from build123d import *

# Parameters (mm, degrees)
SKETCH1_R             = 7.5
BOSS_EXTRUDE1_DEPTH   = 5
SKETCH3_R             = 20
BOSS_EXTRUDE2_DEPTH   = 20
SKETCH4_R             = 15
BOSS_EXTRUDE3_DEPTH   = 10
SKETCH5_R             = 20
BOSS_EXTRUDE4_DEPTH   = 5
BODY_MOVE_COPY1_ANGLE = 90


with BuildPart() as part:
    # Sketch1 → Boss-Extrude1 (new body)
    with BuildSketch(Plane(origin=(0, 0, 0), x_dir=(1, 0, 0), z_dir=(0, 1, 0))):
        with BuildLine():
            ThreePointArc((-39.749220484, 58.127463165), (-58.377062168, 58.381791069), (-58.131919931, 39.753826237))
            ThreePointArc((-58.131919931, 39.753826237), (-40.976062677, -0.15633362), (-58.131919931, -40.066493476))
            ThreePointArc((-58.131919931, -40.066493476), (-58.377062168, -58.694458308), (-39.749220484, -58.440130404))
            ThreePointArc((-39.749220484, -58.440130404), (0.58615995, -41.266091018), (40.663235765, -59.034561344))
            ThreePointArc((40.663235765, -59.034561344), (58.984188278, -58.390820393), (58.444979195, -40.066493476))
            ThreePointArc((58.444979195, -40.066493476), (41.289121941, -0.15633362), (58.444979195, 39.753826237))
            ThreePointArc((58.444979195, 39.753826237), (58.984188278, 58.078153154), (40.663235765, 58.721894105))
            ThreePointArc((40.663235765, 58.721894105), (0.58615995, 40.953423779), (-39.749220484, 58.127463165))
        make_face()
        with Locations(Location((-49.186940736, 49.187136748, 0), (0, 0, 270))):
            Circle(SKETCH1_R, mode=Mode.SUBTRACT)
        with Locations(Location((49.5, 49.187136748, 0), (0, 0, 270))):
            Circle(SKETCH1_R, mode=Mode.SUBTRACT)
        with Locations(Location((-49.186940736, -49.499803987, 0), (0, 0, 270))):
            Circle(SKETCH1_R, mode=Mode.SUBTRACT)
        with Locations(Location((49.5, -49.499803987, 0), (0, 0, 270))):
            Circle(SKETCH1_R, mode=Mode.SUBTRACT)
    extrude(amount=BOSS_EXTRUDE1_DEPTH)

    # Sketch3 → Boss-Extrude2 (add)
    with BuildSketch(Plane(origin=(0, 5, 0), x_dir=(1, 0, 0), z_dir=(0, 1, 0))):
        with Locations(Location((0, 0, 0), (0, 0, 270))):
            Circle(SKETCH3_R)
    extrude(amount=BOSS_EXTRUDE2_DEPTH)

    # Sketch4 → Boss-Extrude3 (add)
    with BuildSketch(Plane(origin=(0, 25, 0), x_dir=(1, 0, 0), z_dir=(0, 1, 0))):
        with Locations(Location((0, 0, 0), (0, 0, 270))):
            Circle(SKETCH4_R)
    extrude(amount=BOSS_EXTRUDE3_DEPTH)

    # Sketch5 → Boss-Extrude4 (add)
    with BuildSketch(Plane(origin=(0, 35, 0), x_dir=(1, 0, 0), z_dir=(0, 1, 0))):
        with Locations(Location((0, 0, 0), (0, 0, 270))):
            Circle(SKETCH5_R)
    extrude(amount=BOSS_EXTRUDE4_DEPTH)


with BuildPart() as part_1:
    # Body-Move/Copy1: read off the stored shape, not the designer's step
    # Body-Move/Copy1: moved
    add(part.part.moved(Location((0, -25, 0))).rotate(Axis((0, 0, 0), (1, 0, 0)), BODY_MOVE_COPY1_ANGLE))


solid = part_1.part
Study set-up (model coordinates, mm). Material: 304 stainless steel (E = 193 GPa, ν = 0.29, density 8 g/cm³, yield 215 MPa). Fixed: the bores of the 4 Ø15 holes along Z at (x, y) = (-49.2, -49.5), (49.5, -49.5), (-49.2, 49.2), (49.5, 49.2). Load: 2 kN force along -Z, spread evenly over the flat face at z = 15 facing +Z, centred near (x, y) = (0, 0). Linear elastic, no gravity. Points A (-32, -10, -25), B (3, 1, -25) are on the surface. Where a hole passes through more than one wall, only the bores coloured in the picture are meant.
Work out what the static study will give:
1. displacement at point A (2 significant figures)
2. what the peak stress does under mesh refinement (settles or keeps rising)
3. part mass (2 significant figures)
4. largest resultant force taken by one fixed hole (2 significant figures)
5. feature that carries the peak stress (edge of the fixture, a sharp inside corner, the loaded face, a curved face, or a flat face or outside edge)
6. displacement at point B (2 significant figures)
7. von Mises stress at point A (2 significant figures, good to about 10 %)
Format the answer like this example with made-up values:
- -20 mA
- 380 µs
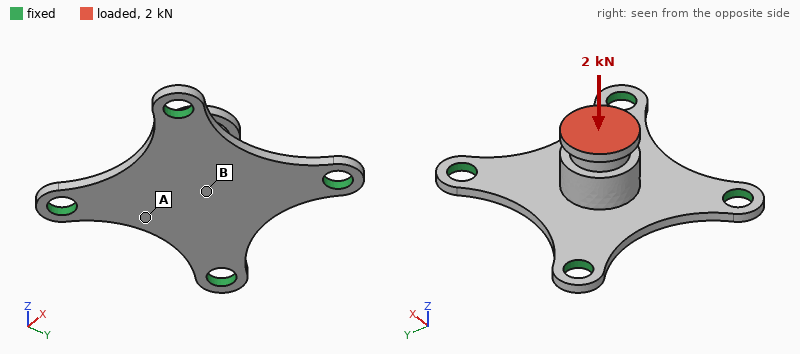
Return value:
- 46 µm
- keeps rising
- 690 g
- 530 N
- edge of the fixture
- 58 µm
- 30 MPa
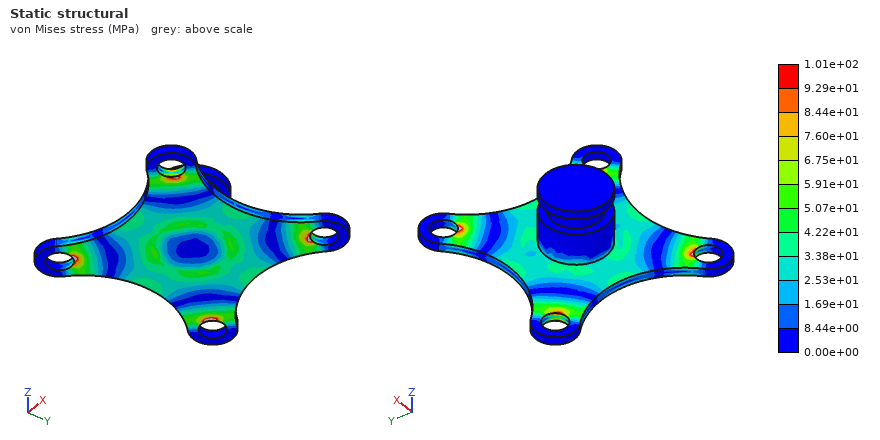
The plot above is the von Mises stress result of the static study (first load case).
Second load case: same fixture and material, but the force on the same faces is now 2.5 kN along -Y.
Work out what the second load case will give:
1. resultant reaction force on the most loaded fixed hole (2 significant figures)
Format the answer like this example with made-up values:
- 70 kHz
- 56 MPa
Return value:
- 1000 N
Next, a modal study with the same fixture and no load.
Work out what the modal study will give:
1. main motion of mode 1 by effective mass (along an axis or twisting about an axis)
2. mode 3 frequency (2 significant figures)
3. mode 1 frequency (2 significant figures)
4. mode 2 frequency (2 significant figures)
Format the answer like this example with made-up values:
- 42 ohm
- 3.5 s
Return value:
- along Z
- 2100 Hz
- 1300 Hz
- 2100 Hz
